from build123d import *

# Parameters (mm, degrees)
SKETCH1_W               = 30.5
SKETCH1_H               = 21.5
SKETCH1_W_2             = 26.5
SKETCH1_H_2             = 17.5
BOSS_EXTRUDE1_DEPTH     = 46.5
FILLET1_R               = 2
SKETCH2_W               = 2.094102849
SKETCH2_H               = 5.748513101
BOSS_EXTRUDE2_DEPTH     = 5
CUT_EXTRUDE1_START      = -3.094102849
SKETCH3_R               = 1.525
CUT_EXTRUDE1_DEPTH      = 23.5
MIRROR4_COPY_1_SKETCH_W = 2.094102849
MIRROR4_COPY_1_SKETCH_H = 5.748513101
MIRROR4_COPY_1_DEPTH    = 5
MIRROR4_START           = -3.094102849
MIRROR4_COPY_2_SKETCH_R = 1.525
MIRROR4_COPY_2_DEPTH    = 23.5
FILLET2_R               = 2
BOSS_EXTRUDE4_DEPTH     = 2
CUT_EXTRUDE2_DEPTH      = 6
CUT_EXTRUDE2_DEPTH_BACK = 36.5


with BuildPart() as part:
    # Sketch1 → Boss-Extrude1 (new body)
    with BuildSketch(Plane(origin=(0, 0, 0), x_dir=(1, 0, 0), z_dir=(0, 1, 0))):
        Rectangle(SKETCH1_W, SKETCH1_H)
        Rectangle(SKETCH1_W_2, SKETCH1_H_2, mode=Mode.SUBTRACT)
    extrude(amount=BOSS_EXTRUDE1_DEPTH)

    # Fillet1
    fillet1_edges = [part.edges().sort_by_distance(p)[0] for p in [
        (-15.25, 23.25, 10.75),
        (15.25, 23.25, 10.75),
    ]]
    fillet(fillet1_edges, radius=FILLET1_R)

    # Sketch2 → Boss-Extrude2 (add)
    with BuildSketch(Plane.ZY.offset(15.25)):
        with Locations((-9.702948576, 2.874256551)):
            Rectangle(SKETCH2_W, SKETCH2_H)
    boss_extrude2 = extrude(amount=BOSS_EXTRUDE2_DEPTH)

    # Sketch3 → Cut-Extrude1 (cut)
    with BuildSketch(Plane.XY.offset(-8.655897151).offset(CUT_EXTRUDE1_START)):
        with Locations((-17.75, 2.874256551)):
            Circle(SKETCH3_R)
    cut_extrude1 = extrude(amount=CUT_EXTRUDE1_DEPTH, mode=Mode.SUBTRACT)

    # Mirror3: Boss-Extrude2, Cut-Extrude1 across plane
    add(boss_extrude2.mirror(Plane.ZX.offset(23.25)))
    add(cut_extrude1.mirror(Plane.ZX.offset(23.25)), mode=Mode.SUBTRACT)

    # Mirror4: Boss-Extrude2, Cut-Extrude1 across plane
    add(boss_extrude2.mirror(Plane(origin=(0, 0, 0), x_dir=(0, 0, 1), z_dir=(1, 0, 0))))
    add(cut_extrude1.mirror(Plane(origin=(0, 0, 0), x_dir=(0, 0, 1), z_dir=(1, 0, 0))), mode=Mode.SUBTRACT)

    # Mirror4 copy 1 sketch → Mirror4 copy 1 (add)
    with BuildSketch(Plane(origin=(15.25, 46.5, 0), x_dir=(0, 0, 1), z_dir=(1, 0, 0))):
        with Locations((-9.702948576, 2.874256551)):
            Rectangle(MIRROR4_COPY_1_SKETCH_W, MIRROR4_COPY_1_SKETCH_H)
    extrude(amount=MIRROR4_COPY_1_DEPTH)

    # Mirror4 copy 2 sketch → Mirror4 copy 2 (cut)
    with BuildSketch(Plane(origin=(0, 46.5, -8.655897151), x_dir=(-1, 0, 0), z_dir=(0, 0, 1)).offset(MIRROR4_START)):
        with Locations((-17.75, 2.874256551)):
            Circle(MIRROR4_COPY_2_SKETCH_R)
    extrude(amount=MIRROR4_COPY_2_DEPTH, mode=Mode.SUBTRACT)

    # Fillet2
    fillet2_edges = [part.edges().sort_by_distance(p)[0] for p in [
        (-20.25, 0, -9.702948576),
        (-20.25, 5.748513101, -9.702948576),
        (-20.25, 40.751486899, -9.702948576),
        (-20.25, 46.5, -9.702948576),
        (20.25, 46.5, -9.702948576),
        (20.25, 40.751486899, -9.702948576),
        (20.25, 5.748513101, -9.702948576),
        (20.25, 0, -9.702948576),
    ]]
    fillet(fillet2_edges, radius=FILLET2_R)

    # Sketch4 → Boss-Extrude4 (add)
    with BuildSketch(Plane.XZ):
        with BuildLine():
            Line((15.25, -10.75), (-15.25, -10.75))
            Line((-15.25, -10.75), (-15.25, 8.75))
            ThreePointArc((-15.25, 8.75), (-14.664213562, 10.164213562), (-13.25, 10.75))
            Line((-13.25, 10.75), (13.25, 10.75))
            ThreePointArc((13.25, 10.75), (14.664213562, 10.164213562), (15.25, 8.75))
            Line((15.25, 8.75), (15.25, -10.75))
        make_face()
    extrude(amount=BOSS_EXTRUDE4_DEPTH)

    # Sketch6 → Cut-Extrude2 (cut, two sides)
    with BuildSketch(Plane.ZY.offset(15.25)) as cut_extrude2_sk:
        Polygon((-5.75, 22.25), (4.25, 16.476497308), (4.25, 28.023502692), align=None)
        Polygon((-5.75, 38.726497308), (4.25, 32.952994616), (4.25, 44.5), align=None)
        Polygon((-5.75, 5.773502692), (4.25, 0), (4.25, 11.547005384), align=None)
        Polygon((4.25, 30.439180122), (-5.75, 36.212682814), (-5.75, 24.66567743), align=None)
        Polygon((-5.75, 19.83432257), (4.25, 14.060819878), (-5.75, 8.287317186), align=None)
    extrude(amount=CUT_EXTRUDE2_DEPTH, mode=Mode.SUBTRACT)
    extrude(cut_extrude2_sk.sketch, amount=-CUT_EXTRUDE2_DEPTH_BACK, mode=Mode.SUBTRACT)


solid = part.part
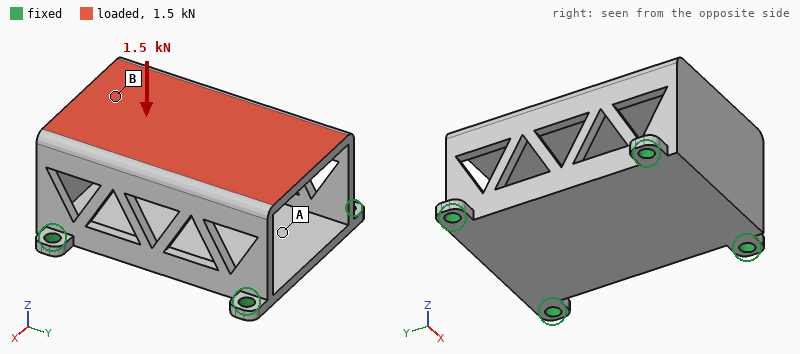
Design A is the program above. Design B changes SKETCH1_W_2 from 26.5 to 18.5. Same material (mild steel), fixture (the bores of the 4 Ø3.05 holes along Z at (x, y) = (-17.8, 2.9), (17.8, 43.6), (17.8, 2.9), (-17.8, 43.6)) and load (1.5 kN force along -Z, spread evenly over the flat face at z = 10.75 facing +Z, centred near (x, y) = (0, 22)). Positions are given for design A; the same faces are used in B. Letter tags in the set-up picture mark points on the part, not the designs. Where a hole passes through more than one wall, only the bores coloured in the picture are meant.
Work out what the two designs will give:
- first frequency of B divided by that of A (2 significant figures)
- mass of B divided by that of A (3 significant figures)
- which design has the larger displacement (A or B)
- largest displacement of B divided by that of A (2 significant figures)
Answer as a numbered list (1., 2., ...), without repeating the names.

1. 1.3
2. 1.46
3. A
4. 0.22
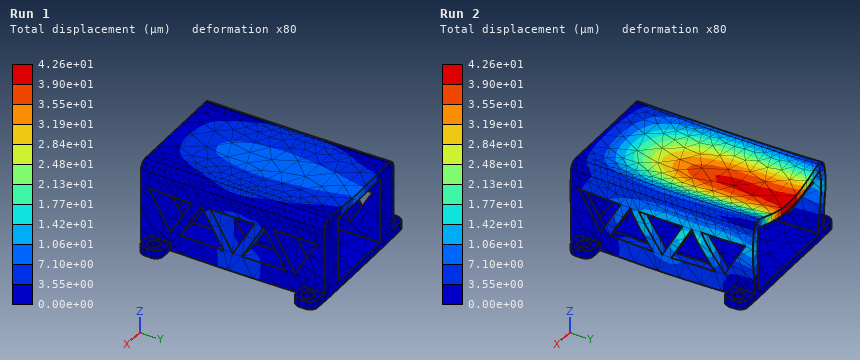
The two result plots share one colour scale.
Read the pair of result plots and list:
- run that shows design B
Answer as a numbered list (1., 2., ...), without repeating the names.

1. Run 1
